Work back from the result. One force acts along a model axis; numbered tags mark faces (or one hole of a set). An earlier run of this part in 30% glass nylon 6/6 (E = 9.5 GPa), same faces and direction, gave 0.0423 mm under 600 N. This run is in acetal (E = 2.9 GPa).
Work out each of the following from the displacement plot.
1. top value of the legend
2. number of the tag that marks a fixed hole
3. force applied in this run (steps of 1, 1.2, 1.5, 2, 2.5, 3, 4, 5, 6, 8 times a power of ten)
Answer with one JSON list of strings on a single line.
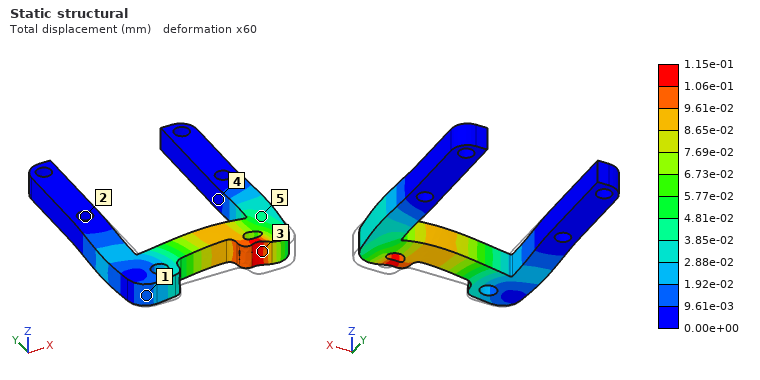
["1.15e-01 mm", "2", "500 N"]
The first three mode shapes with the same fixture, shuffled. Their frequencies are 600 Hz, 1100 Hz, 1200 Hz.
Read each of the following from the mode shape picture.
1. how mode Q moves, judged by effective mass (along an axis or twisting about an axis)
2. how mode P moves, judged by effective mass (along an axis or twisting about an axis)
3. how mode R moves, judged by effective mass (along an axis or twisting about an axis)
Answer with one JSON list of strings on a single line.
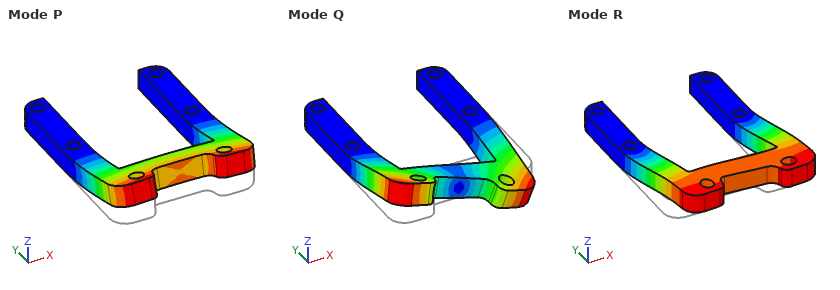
["twisting about Y", "along Z", "along X"]
